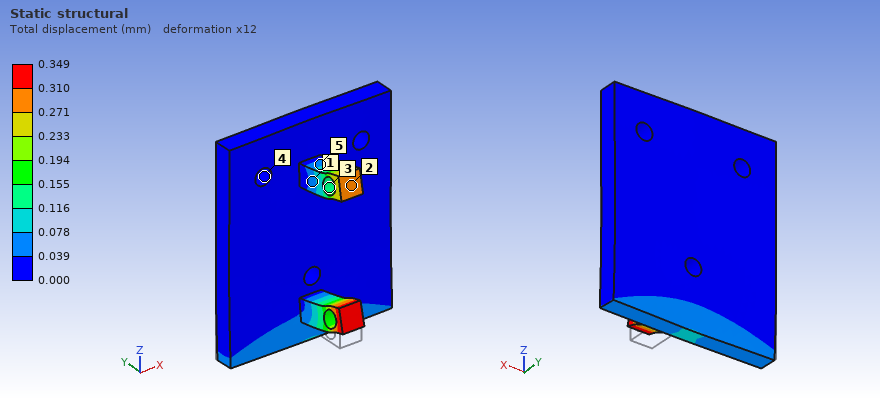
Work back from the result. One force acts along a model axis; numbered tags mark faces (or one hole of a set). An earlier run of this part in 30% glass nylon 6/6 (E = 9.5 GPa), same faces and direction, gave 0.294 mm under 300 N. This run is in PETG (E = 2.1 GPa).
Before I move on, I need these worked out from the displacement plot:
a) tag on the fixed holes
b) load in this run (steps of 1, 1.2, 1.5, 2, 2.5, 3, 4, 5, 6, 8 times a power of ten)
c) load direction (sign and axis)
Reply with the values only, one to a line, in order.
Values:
4
80 N
+Z
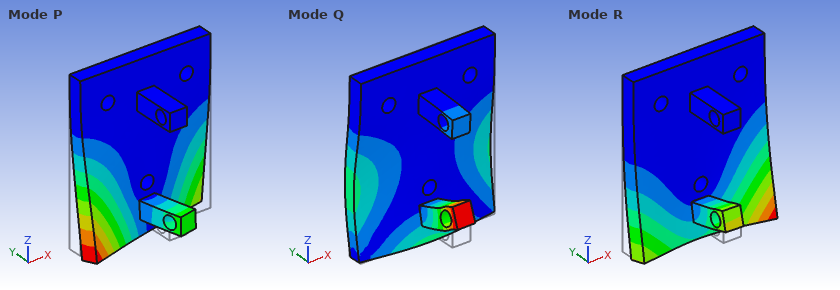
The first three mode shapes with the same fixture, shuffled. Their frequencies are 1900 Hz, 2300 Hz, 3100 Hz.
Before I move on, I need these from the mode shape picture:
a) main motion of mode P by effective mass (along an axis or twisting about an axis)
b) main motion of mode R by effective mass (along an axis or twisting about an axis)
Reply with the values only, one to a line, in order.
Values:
twisting about Z
along Y
